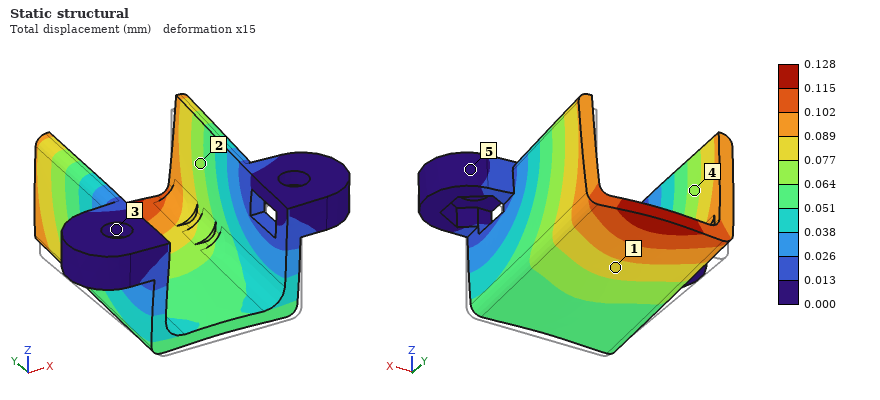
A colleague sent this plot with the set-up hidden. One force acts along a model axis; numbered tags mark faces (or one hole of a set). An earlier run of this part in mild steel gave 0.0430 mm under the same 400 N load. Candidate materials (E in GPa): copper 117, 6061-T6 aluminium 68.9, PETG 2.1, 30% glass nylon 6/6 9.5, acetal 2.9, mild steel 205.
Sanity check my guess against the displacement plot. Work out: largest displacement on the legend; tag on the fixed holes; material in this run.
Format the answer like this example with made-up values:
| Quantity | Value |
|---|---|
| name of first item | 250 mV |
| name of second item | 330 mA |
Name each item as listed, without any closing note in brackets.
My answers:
| Quantity | Value |
|---|---|
| largest displacement on the legend | 0.128 mm |
| tag on the fixed holes | 3 |
| material in this run | 6061-T6 aluminium |
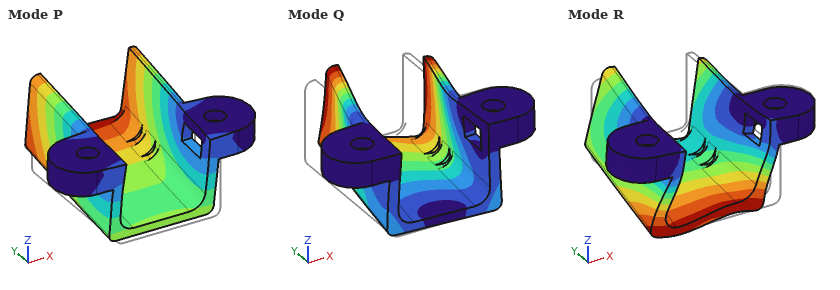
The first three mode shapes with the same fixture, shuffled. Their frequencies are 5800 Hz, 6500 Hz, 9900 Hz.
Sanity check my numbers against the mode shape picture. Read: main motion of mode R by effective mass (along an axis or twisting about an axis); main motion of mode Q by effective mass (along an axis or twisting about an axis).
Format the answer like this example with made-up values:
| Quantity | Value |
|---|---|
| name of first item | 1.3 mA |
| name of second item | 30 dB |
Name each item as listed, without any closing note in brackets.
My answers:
| Quantity | Value |
|---|---|
| main motion of mode R by effective mass | along X |
| main motion of mode Q by effective mass | along X |
